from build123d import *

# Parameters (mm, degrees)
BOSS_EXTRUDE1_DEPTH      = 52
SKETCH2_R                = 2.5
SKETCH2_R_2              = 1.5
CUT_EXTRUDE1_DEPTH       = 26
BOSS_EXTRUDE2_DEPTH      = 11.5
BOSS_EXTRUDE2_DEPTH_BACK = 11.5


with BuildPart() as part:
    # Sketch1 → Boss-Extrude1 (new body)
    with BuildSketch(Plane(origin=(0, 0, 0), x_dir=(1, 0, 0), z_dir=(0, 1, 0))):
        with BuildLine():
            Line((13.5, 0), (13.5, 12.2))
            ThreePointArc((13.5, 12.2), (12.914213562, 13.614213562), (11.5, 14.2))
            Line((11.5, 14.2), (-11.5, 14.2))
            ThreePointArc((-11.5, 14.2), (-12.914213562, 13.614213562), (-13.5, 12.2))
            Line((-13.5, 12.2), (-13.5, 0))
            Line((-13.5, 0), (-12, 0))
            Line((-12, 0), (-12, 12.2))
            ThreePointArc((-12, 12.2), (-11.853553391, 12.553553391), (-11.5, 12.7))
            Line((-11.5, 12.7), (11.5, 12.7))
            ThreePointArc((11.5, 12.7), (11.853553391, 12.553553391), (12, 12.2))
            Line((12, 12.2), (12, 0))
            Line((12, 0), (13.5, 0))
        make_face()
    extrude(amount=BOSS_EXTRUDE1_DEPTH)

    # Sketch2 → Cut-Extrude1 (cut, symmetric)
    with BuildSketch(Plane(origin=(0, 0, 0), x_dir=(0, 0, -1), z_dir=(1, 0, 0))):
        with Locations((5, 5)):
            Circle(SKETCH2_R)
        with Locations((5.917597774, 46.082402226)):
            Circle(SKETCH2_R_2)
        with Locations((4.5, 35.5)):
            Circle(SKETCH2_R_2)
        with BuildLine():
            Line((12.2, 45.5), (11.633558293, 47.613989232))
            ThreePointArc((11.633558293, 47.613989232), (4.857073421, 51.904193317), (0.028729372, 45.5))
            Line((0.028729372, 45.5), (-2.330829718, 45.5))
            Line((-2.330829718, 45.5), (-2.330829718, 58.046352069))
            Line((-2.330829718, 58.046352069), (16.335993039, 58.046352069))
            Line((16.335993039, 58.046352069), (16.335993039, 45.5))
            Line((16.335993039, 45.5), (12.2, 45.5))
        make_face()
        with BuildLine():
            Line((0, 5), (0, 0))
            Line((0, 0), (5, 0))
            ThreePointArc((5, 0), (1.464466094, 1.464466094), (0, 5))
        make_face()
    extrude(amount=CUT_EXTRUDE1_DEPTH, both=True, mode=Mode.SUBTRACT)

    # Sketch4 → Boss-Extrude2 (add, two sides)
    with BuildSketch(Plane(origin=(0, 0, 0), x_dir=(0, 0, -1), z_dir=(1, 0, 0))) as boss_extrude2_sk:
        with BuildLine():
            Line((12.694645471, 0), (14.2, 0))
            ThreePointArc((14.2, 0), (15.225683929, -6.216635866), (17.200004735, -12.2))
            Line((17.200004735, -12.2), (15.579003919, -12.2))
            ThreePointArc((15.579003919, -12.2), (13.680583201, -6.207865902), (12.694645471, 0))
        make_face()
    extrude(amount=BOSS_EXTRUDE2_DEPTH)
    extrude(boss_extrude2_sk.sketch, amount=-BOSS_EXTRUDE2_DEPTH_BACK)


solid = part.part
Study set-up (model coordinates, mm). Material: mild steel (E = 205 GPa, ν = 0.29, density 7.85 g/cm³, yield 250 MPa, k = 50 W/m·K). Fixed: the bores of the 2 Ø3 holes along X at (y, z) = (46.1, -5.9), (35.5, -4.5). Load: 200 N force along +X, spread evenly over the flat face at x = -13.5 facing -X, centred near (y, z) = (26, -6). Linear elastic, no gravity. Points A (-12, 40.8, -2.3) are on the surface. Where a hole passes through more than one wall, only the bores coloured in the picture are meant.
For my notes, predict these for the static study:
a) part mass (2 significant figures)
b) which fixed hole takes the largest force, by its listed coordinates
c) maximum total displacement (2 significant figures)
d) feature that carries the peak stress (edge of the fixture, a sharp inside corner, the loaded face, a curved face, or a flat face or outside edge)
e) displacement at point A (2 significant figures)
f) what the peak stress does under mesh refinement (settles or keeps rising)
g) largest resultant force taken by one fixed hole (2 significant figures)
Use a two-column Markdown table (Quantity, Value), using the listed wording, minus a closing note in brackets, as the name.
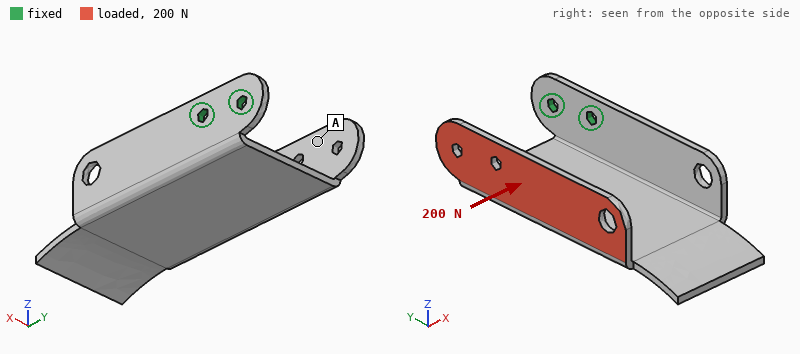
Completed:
| Quantity | Value |
|---|---|
| part mass | 31 g |
| which fixed hole takes the largest force, by its listed coordinates | (35.5, -4.5) |
| maximum total displacement | 0.38 mm |
| feature that carries the peak stress | edge of the fixture |
| displacement at point A | 0.27 mm |
| what the peak stress does under mesh refinement | keeps rising |
| largest resultant force taken by one fixed hole | 290 N |
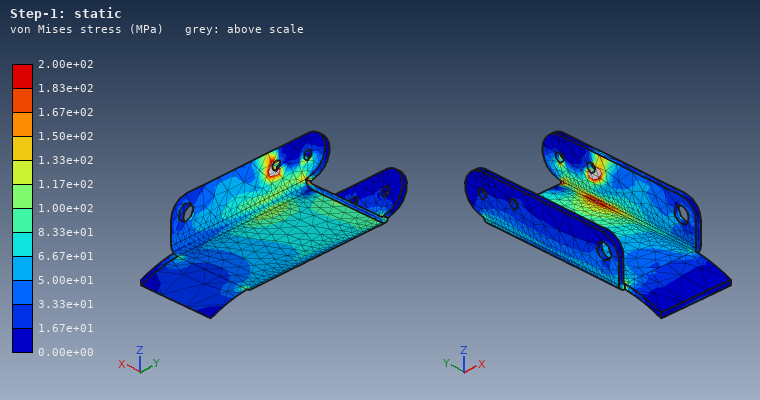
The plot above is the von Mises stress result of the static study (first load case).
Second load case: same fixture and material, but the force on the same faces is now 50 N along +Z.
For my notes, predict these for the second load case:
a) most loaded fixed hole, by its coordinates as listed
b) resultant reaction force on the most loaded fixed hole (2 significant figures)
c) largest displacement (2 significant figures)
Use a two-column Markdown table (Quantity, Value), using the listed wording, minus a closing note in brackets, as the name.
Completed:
| Quantity | Value |
|---|---|
| most loaded fixed hole, by its coordinates as listed | (35.5, -4.5) |
| resultant reaction force on the most loaded fixed hole | 80 N |
| largest displacement | 0.37 mm |
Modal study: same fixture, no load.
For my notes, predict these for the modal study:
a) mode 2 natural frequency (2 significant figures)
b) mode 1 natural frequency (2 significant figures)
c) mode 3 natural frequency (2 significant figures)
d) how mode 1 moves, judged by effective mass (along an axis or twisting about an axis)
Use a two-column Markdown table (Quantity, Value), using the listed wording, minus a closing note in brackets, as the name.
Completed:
| Quantity | Value |
|---|---|
| mode 2 natural frequency | 860 Hz |
| mode 1 natural frequency | 520 Hz |
| mode 3 natural frequency | 1300 Hz |
| how mode 1 moves, judged by effective mass | along Z |
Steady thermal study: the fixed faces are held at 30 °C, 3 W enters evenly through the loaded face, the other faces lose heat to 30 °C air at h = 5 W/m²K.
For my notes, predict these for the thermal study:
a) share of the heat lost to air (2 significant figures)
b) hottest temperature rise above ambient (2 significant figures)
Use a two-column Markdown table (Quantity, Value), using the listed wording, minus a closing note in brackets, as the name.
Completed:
| Quantity | Value |
|---|---|
| share of the heat lost to air | 21 % |
| hottest temperature rise above ambient | 43 K |
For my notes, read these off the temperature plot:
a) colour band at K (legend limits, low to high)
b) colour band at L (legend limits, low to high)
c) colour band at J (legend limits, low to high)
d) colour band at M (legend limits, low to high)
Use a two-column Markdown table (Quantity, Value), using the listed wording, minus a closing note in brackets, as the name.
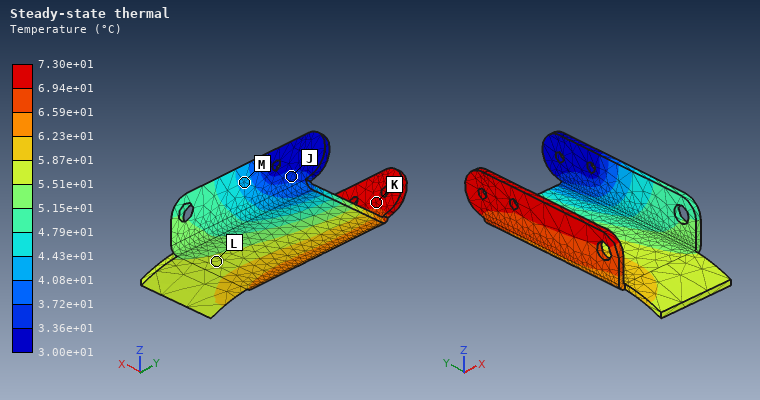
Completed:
| Quantity | Value |
|---|---|
| colour band at K | 6.94e+01 to 7.30e+01 °C |
| colour band at L | 5.51e+01 to 5.87e+01 °C |
| colour band at J | 3.36e+01 to 3.72e+01 °C |
| colour band at M | 4.08e+01 to 4.43e+01 °C |
